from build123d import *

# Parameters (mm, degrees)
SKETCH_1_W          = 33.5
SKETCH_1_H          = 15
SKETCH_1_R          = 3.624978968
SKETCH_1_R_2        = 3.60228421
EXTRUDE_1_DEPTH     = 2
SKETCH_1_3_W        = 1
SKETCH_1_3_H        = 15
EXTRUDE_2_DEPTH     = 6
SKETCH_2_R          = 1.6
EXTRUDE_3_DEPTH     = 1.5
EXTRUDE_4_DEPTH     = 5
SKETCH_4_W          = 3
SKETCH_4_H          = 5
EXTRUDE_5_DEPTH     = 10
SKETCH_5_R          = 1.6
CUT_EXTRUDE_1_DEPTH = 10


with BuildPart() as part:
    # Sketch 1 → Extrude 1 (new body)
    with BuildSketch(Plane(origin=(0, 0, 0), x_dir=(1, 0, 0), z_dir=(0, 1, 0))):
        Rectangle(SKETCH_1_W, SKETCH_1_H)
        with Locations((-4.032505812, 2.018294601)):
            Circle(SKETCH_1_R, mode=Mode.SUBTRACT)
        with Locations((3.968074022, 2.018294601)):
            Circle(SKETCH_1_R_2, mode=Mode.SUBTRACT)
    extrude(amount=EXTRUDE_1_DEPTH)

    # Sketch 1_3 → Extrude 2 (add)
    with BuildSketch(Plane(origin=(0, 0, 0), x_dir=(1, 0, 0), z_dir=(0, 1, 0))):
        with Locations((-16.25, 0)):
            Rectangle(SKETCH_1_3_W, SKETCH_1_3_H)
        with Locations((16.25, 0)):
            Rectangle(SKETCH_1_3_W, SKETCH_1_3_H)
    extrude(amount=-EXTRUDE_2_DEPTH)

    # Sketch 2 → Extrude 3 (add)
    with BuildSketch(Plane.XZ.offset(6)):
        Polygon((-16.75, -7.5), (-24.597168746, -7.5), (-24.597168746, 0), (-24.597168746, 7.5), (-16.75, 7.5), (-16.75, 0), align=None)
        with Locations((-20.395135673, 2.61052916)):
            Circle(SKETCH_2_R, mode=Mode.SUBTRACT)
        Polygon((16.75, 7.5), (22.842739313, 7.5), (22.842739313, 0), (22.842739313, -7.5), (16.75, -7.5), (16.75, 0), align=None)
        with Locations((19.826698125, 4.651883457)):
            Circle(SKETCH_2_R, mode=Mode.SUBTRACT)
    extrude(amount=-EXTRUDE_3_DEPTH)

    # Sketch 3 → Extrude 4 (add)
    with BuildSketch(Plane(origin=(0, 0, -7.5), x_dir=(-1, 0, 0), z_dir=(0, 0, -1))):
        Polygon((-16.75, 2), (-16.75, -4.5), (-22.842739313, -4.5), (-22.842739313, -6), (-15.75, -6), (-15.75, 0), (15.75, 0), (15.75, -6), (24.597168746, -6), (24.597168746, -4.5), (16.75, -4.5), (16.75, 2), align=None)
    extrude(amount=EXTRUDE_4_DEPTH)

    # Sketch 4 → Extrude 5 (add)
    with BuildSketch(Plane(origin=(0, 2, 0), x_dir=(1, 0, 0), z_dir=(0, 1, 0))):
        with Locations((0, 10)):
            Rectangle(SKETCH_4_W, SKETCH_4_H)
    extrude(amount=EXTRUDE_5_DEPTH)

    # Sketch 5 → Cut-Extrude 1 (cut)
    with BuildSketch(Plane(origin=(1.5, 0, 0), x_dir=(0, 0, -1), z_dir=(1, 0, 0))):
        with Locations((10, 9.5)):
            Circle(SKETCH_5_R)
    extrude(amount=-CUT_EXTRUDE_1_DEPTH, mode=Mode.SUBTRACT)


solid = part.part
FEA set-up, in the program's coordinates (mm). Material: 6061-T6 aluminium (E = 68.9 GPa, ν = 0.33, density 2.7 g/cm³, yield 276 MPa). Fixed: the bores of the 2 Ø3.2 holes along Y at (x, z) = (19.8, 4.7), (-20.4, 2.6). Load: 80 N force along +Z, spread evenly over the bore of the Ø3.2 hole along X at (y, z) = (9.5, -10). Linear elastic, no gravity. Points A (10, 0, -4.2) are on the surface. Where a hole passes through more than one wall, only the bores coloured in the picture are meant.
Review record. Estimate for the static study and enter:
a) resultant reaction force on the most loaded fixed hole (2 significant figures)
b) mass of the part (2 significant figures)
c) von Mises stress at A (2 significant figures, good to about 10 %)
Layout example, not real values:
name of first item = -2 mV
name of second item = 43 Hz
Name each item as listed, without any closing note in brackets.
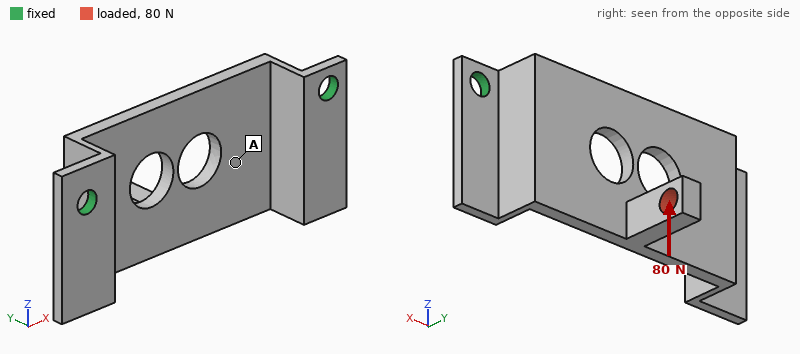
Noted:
resultant reaction force on the most loaded fixed hole = 43 N
mass of the part = 5.2 g
von Mises stress at A = 27 MPa
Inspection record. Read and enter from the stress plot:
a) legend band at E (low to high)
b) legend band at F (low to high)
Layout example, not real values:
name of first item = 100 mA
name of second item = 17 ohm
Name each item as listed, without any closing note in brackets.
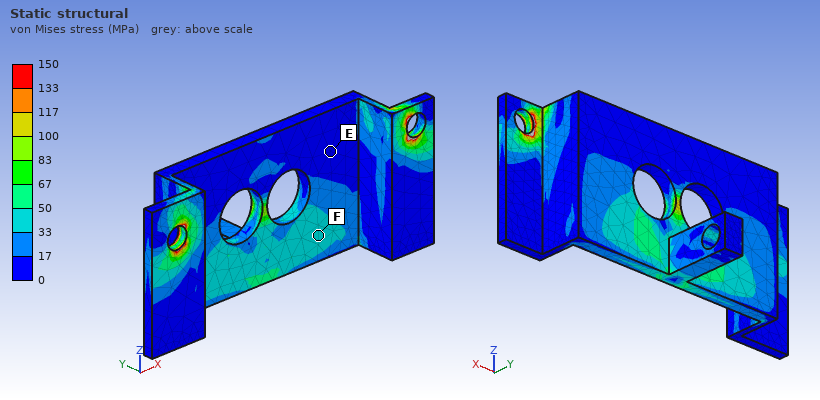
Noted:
legend band at E = 0 to 17 MPa
legend band at F = 33 to 50 MPa
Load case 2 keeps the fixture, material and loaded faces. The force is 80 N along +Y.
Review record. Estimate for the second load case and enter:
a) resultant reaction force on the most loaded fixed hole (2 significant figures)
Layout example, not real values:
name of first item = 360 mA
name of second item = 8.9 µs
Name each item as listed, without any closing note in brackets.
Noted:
resultant reaction force on the most loaded fixed hole = 70 N
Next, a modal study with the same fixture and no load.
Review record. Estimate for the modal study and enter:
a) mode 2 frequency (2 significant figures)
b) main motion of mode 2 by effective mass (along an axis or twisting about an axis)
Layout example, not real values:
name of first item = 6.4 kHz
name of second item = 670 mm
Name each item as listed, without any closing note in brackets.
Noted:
mode 2 frequency = 6100 Hz
main motion of mode 2 by effective mass = along X
